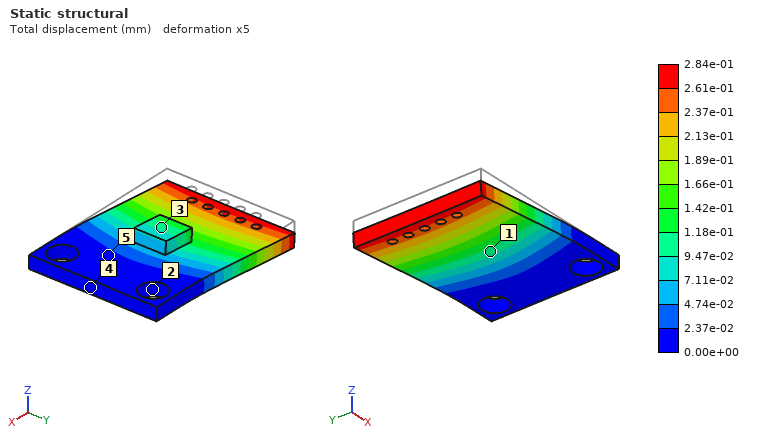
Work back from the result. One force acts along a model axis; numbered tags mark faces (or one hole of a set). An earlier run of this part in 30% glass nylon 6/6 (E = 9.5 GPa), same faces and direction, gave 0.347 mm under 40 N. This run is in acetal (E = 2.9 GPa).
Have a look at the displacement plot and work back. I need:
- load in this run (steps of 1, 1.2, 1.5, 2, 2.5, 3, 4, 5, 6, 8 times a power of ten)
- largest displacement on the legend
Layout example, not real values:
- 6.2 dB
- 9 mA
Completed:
- 10 N
- 2.84e-01 mm
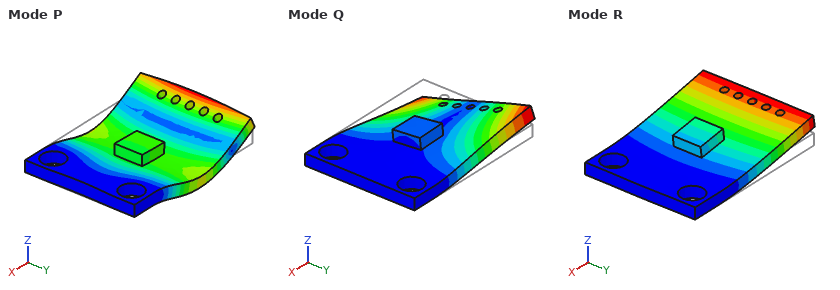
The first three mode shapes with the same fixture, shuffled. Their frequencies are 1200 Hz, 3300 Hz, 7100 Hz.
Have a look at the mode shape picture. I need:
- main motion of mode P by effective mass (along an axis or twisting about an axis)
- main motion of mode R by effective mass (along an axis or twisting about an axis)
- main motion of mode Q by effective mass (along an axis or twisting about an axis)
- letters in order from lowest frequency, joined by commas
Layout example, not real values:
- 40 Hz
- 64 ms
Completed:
- along Z
- along Z
- twisting about X
- R, Q, P
